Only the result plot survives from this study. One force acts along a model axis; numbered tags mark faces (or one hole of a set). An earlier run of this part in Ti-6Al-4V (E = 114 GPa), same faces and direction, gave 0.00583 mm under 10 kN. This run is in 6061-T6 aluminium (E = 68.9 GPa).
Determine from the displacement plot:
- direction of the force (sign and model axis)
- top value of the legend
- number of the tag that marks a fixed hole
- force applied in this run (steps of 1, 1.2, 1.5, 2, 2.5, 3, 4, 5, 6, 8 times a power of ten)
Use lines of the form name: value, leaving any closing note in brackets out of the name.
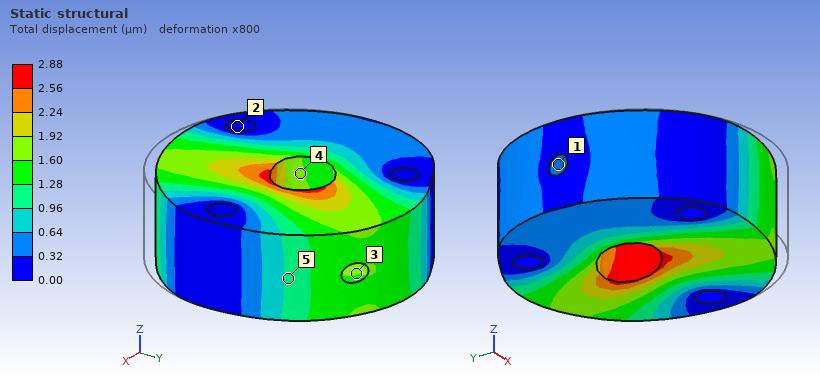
direction of the force: +Y
top value of the legend: 2.88 µm
number of the tag that marks a fixed hole: 2
force applied in this run: 3 kN
